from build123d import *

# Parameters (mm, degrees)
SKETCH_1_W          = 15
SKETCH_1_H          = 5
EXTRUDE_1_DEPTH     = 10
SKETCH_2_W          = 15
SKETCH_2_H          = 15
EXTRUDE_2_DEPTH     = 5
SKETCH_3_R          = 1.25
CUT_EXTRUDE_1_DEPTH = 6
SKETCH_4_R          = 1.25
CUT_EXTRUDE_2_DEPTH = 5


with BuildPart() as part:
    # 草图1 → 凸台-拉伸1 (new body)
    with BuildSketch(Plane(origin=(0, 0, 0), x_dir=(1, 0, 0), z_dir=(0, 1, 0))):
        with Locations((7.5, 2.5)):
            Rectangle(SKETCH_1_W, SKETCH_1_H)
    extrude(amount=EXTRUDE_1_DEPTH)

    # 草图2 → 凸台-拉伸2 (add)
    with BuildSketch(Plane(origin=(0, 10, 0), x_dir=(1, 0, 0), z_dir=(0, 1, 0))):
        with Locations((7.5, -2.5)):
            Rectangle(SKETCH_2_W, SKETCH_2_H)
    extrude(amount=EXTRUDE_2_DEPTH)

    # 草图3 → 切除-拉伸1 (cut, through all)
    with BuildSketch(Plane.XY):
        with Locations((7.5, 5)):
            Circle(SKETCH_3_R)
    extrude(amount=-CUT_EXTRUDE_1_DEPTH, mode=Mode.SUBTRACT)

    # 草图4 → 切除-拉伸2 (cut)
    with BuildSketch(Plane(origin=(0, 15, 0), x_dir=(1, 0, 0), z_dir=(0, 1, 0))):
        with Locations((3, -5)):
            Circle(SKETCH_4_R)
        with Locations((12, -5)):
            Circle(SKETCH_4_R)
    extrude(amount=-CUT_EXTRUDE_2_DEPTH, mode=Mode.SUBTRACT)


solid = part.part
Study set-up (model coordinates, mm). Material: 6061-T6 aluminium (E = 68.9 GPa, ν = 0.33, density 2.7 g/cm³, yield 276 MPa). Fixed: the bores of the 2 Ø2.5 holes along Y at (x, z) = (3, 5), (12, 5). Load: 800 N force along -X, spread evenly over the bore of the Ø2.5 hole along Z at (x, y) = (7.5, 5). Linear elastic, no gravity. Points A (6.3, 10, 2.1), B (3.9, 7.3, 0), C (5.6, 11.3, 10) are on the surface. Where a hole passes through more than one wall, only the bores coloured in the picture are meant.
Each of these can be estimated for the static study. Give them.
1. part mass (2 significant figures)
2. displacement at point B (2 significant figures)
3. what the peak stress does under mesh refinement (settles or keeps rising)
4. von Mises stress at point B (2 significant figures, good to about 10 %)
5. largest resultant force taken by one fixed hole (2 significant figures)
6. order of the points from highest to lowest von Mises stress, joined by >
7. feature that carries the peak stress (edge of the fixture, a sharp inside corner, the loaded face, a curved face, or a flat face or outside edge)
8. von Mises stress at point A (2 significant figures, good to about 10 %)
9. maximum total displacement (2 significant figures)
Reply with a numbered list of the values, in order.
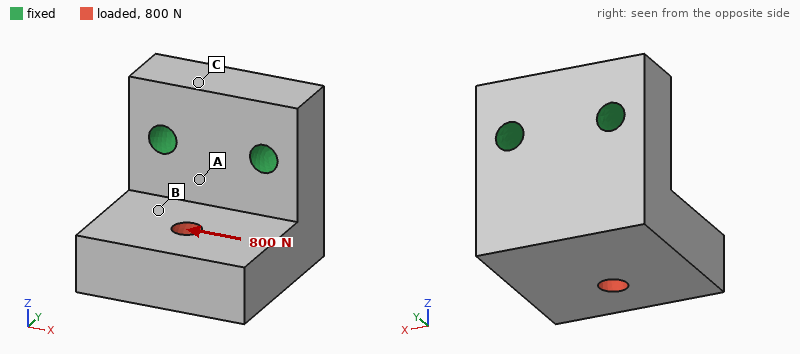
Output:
1. 4.9 g
2. 14 µm
3. keeps rising
4. 35 MPa
5. 830 N
6. A > B > C
7. edge of the fixture
8. 66 MPa
9. 29 µm
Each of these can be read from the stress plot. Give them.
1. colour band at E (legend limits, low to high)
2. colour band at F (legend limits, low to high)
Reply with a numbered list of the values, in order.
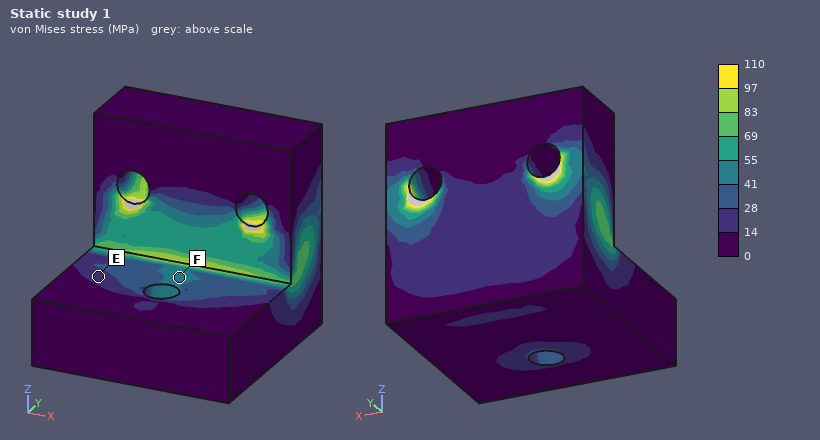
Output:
1. 14 to 28 MPa
2. 41 to 55 MPa
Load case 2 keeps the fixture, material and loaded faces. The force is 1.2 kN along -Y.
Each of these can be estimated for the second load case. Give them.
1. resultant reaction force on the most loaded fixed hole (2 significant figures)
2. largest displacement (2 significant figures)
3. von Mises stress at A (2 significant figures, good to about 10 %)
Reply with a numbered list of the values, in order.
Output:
1. 600 N
2. 50 µm
3. 63 MPa
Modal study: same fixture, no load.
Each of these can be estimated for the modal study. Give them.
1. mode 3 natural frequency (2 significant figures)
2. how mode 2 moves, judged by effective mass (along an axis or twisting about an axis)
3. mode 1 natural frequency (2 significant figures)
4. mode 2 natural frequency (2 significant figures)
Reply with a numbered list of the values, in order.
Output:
1. 36 kHz
2. along X
3. 13 kHz
4. 21 kHz
